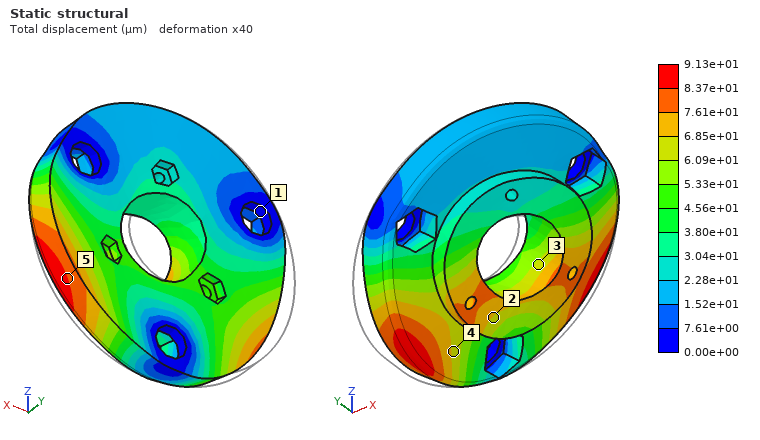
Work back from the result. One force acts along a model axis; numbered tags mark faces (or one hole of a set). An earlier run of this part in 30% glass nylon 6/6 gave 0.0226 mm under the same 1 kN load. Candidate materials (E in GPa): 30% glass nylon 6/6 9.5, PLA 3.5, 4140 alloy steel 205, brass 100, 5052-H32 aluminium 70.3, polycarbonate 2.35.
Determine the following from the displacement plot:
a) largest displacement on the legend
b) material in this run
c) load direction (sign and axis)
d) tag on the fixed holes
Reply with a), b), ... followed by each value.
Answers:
a) 9.13e+01 µm
b) polycarbonate
c) +X
d) 1
